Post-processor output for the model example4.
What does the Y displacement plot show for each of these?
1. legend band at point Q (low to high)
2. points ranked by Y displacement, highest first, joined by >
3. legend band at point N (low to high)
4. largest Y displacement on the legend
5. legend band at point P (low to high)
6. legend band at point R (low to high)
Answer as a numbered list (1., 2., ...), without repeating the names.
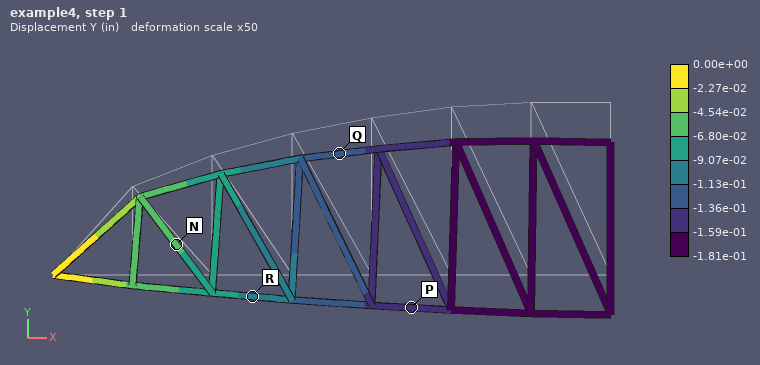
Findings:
1. -1.36e-01 to -1.13e-01 in
2. N > R > Q > P
3. -6.80e-02 to -4.54e-02 in
4. 0.00e+00 in
5. -1.59e-01 to -1.36e-01 in
6. -1.13e-01 to -9.07e-02 in
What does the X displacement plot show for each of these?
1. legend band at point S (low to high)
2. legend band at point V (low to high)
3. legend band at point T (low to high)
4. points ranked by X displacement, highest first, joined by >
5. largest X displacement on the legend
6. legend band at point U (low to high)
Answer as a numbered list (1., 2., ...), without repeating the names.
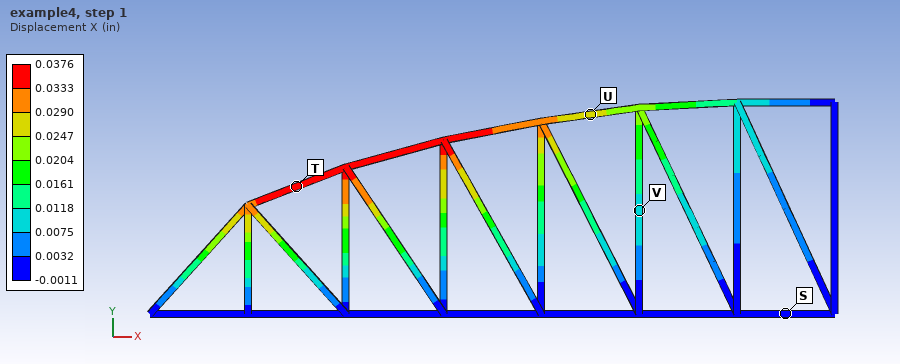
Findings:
1. -0.0011 to 0.0032 in
2. 0.0075 to 0.0118 in
3. 0.0333 to 0.0376 in
4. T > U > V > S
5. 0.0376 in
6. 0.0247 to 0.0290 in
